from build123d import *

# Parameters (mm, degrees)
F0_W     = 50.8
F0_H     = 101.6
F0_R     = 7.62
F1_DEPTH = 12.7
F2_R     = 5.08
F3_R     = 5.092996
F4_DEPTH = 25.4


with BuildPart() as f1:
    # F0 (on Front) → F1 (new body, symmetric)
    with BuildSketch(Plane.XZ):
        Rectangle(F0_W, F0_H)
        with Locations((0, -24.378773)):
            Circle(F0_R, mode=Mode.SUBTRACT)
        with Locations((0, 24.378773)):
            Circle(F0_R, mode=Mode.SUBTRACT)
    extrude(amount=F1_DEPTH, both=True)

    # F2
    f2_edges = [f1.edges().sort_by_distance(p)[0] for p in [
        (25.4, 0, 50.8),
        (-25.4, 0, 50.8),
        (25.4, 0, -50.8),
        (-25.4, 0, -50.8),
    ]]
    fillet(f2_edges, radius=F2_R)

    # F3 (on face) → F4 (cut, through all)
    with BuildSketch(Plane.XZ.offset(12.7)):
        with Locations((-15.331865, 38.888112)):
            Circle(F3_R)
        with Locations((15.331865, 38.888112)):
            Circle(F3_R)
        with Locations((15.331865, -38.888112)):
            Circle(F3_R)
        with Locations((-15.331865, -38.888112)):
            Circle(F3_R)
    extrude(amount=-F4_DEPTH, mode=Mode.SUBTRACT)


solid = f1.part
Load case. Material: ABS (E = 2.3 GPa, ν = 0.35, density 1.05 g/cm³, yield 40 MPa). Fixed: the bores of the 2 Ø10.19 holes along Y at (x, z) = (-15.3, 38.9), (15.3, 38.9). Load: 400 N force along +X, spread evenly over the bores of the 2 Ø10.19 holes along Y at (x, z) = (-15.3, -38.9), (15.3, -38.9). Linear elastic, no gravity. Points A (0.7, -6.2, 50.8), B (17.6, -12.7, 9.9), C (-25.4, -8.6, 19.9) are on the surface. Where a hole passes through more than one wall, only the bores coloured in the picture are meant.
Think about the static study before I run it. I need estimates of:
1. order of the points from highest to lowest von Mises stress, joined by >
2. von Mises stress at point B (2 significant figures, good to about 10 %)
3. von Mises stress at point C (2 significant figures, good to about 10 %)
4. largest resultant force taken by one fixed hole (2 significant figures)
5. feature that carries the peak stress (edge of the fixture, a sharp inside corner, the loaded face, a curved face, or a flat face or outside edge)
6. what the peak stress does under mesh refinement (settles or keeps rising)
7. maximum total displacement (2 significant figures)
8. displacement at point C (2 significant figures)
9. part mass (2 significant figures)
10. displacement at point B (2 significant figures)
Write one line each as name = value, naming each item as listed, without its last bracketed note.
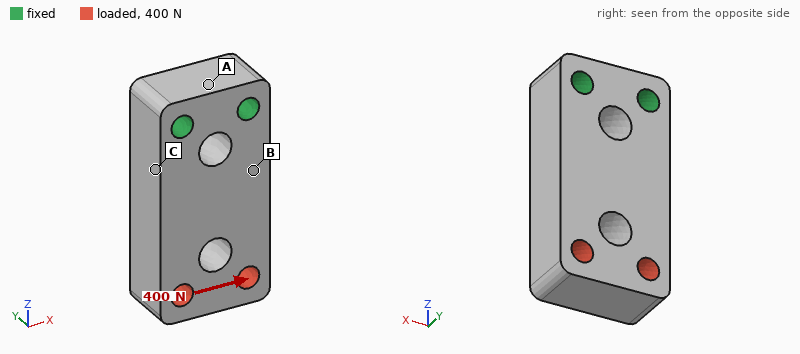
order of the points from highest to lowest von Mises stress, joined by > = C > B > A
von Mises stress at point B = 1.2 MPa
von Mises stress at point C = 1.8 MPa
largest resultant force taken by one fixed hole = 820 N
feature that carries the peak stress = edge of the fixture
what the peak stress does under mesh refinement = keeps rising
maximum total displacement = 0.17 mm
displacement at point C = 0.033 mm
part mass = 120 g
displacement at point B = 0.041 mm
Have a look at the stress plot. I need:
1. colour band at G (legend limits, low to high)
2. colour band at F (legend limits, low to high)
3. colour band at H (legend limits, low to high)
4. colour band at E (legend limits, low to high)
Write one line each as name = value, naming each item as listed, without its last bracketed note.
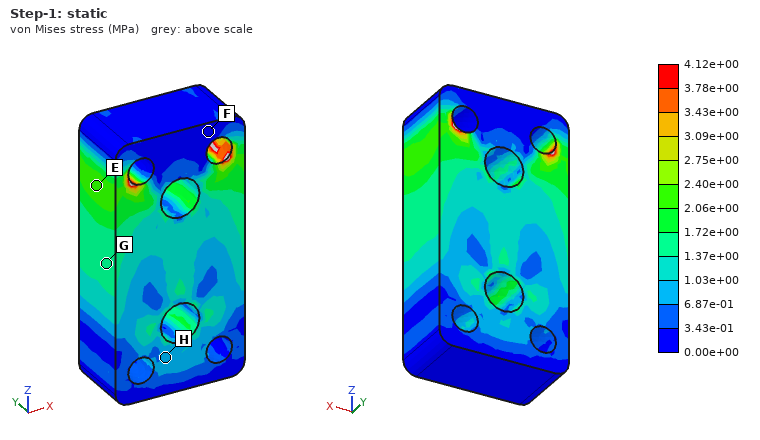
colour band at G = 1.37e+00 to 1.72e+00 MPa
colour band at F = 0.00e+00 to 3.43e-01 MPa
colour band at H = 6.87e-01 to 1.03e+00 MPa
colour band at E = 2.06e+00 to 2.40e+00 MPa
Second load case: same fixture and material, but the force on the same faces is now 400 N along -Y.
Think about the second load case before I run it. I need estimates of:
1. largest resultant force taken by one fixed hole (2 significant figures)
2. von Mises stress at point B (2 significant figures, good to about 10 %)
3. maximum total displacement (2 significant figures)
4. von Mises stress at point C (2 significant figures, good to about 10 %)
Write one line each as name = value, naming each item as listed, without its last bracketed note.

largest resultant force taken by one fixed hole = 200 N
von Mises stress at point B = 4.2 MPa
maximum total displacement = 0.59 mm
von Mises stress at point C = 3.3 MPa
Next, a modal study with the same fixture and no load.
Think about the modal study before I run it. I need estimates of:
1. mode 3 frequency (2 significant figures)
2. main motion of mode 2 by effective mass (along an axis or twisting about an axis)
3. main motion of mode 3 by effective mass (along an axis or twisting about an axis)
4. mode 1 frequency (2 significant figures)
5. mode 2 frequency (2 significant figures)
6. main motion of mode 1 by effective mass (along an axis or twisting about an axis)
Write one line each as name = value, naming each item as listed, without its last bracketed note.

mode 3 frequency = 2000 Hz
main motion of mode 2 by effective mass = along X
main motion of mode 3 by effective mass = twisting about Z
mode 1 frequency = 740 Hz
mode 2 frequency = 1300 Hz
main motion of mode 1 by effective mass = along Y
